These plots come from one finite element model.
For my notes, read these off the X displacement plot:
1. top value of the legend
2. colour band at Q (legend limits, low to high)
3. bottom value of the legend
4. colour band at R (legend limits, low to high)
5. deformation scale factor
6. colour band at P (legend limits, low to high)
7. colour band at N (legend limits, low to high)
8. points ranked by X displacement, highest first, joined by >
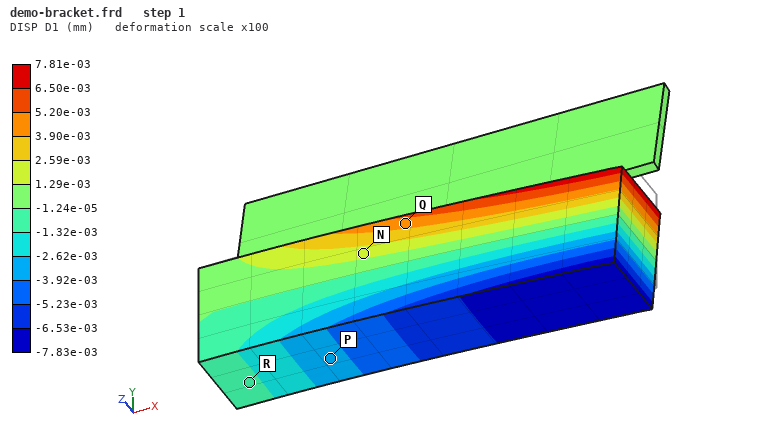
7.81e-03 mm
3.90e-03 to 5.20e-03 mm
-7.83e-03 mm
-1.32e-03 to -1.24e-05 mm
100
-3.92e-03 to -2.62e-03 mm
1.29e-03 to 2.59e-03 mm
Q > N > R > P
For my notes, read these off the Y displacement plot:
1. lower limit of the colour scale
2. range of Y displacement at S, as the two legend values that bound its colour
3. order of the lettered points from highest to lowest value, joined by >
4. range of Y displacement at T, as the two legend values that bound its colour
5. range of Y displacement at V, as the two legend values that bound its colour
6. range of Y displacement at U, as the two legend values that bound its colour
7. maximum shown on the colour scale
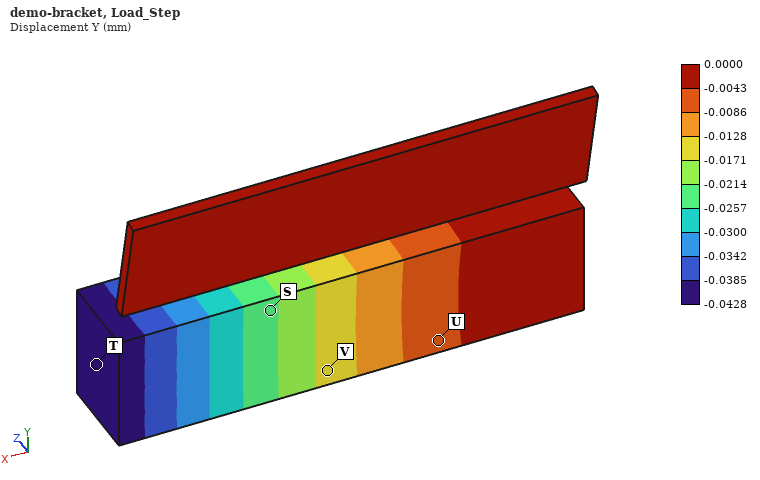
-0.0428 mm
-0.0257 to -0.0214 mm
U > V > S > T
-0.0428 to -0.0385 mm
-0.0171 to -0.0128 mm
-0.0086 to -0.0043 mm
0.0000 mm
